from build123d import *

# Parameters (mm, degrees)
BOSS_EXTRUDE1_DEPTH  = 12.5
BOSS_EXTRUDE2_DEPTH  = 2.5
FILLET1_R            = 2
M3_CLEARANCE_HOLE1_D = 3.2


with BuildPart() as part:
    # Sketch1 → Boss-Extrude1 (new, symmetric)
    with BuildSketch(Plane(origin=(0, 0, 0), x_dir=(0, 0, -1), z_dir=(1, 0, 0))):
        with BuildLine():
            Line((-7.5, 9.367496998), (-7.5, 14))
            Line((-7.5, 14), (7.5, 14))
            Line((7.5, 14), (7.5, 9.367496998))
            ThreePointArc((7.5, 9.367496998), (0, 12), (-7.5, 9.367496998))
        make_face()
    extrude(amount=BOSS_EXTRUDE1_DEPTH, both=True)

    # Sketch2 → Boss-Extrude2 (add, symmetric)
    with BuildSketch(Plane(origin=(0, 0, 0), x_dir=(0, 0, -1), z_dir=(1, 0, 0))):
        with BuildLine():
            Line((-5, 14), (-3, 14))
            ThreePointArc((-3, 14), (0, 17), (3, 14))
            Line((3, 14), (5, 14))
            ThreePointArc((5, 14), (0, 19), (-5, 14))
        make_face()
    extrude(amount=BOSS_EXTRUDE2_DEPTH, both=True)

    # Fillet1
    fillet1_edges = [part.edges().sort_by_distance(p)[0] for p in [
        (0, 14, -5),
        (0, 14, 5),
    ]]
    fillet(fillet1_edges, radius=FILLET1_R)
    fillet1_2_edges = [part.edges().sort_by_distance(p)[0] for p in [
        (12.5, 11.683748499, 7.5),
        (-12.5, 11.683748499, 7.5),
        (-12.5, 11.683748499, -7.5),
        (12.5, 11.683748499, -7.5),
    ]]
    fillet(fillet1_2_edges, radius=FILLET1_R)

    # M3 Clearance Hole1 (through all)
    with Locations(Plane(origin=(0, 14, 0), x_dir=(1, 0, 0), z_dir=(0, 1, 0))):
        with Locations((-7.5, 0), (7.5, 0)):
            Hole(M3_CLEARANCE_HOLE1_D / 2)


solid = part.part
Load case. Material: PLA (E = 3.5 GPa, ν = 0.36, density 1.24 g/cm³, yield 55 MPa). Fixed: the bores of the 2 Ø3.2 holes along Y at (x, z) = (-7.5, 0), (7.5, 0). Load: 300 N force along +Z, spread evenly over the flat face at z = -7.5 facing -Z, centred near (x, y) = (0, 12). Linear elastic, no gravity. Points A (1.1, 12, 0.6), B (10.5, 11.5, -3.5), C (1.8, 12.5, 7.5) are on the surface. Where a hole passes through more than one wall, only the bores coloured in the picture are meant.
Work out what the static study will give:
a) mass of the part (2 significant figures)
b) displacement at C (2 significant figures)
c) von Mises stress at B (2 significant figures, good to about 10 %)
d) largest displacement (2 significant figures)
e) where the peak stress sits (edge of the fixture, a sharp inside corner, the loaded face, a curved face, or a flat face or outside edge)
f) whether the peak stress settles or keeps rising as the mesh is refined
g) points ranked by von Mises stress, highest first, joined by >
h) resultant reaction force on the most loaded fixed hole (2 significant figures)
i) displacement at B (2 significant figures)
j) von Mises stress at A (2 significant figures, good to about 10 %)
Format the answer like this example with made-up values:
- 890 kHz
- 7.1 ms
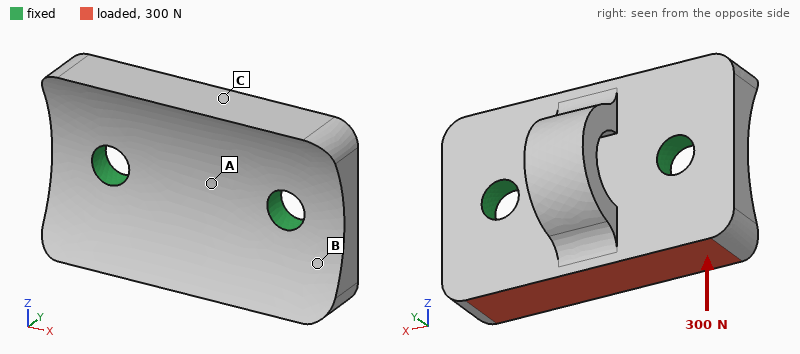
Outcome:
- 1.4 g
- 0.028 mm
- 12 MPa
- 0.13 mm
- edge of the fixture
- keeps rising
- B > A > C
- 150 N
- 0.027 mm
- 8.3 MPa
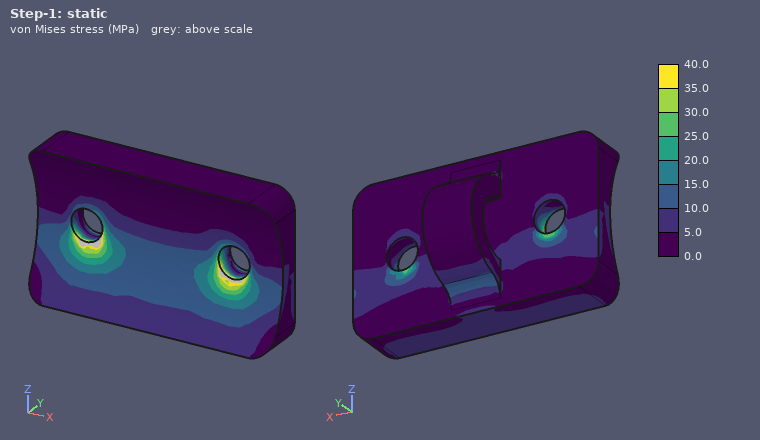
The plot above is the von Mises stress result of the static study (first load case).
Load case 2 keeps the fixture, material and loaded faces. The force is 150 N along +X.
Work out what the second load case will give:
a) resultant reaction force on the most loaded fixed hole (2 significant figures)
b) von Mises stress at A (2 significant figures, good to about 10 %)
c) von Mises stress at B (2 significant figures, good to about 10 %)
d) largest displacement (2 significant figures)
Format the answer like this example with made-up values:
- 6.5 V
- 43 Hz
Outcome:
- 97 N
- 2.5 MPa
- 2.8 MPa
- 27 µm
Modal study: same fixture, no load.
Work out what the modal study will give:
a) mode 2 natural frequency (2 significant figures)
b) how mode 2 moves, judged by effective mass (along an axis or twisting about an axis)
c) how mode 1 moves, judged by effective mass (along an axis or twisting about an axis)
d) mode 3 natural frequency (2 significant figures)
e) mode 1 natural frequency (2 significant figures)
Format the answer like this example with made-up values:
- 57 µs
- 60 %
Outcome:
- 9400 Hz
- along Y
- twisting about X
- 12 kHz
- 7300 Hz
